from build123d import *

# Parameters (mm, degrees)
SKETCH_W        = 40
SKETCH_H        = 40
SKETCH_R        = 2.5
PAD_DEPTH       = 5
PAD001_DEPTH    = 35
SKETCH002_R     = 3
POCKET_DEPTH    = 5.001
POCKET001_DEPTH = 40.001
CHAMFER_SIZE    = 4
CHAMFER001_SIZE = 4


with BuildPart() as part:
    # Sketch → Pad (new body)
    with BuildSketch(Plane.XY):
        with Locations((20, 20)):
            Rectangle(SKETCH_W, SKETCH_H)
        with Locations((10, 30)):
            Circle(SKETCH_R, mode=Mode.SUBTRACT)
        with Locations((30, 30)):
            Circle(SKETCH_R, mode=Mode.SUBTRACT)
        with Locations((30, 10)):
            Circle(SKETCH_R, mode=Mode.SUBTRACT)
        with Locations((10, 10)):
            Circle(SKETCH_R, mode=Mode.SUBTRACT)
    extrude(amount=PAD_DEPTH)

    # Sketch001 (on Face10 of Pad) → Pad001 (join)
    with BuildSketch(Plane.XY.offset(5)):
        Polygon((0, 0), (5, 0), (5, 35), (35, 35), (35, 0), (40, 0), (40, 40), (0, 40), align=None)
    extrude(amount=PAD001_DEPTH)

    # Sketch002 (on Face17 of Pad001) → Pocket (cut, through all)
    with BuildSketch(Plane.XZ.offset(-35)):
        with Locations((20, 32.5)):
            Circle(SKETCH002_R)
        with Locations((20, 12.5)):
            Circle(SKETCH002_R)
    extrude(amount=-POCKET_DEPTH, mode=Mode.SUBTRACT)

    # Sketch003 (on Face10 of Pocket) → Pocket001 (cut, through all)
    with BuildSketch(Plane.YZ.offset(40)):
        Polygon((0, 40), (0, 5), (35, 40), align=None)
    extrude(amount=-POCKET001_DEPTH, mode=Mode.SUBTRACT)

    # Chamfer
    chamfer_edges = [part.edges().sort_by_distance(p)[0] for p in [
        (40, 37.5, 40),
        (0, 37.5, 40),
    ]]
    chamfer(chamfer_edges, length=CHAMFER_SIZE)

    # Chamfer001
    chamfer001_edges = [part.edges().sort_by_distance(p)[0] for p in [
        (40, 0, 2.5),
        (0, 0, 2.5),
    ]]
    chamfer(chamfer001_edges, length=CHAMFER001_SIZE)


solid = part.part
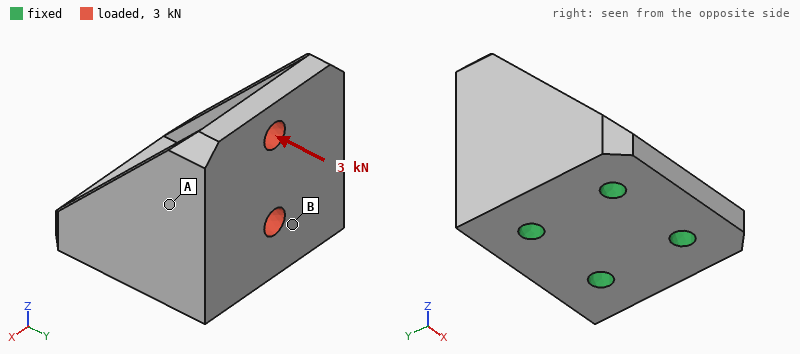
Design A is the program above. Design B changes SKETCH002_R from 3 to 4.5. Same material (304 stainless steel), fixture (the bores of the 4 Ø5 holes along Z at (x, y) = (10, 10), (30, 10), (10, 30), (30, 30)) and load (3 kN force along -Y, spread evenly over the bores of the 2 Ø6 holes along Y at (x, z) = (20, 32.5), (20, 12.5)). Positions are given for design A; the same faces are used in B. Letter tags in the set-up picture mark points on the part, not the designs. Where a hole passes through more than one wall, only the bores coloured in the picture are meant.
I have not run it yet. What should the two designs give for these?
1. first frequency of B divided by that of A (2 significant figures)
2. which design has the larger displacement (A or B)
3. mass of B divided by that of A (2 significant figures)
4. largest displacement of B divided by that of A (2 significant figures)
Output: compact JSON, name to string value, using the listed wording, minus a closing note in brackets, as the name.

{"first frequency of B divided by that of A": "0.98", "which design has the larger displacement": "B", "mass of B divided by that of A": "0.98", "largest displacement of B divided by that of A": "1.1"}
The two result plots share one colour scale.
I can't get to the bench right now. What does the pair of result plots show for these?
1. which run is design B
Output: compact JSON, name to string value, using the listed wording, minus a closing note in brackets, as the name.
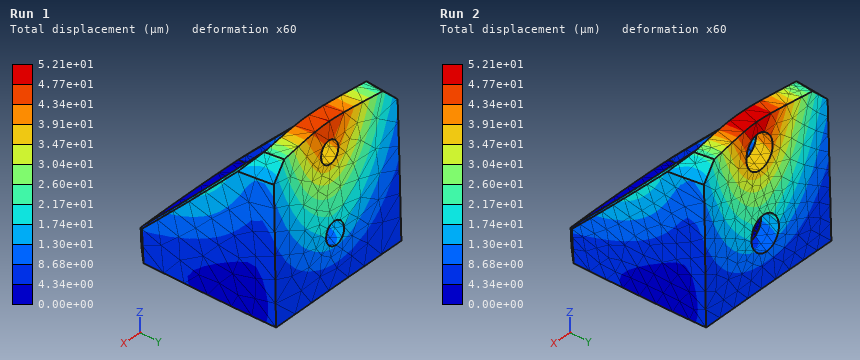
{"which run is design B": "Run 2"}
